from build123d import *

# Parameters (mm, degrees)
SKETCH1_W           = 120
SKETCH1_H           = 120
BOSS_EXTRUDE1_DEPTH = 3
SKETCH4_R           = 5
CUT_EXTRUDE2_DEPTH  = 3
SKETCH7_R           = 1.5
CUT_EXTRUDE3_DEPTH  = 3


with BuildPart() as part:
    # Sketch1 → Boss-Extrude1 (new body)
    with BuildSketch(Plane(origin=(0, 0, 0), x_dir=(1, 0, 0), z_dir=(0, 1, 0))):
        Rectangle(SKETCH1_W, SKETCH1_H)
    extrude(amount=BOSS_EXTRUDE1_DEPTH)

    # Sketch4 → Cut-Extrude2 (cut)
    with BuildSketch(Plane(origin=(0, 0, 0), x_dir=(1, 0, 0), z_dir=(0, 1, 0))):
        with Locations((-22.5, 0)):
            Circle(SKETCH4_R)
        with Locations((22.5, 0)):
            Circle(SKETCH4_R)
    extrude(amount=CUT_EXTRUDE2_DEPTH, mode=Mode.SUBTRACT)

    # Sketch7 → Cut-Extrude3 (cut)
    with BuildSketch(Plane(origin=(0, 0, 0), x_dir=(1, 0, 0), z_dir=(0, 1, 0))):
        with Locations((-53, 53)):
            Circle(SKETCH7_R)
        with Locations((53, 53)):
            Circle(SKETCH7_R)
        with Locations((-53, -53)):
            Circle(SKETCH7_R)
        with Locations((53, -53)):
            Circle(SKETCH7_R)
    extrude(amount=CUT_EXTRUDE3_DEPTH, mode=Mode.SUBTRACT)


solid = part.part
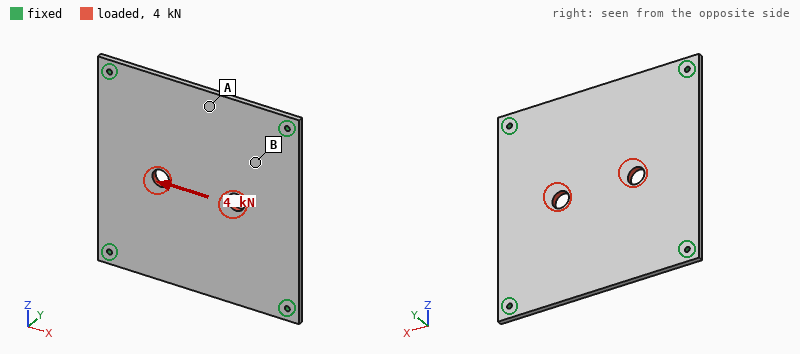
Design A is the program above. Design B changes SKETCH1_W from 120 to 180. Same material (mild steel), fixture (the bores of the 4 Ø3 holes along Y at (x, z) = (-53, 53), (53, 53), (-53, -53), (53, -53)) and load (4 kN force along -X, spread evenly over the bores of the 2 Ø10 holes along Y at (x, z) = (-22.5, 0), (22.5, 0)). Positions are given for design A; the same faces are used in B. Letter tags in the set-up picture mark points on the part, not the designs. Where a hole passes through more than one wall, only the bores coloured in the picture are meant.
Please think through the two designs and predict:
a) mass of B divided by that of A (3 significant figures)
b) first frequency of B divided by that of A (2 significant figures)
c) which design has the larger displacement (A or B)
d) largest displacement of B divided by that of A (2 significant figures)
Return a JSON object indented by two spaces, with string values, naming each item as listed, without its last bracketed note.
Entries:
{
  "mass of B divided by that of A": "1.51",
  "first frequency of B divided by that of A": "1.0",
  "which design has the larger displacement": "A",
  "largest displacement of B divided by that of A": "0.79"
}
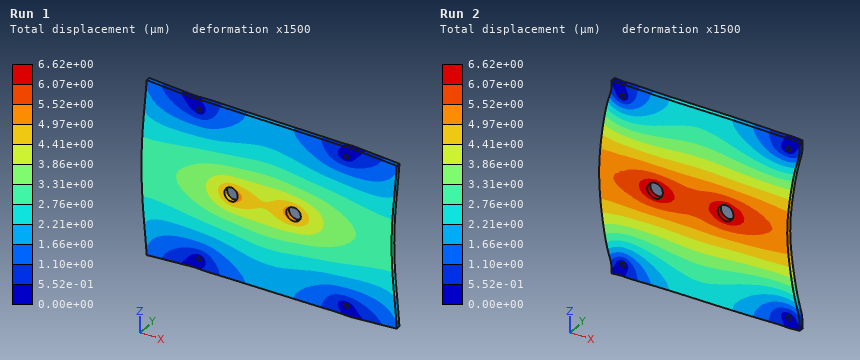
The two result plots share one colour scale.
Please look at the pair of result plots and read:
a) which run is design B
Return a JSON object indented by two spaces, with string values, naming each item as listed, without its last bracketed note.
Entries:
{
  "which run is design B": "Run 1"
}
